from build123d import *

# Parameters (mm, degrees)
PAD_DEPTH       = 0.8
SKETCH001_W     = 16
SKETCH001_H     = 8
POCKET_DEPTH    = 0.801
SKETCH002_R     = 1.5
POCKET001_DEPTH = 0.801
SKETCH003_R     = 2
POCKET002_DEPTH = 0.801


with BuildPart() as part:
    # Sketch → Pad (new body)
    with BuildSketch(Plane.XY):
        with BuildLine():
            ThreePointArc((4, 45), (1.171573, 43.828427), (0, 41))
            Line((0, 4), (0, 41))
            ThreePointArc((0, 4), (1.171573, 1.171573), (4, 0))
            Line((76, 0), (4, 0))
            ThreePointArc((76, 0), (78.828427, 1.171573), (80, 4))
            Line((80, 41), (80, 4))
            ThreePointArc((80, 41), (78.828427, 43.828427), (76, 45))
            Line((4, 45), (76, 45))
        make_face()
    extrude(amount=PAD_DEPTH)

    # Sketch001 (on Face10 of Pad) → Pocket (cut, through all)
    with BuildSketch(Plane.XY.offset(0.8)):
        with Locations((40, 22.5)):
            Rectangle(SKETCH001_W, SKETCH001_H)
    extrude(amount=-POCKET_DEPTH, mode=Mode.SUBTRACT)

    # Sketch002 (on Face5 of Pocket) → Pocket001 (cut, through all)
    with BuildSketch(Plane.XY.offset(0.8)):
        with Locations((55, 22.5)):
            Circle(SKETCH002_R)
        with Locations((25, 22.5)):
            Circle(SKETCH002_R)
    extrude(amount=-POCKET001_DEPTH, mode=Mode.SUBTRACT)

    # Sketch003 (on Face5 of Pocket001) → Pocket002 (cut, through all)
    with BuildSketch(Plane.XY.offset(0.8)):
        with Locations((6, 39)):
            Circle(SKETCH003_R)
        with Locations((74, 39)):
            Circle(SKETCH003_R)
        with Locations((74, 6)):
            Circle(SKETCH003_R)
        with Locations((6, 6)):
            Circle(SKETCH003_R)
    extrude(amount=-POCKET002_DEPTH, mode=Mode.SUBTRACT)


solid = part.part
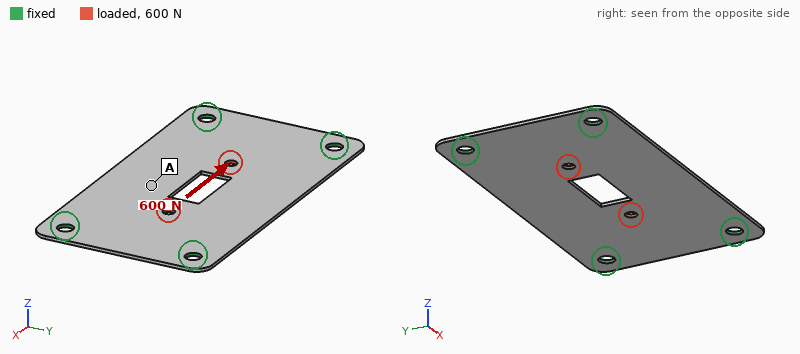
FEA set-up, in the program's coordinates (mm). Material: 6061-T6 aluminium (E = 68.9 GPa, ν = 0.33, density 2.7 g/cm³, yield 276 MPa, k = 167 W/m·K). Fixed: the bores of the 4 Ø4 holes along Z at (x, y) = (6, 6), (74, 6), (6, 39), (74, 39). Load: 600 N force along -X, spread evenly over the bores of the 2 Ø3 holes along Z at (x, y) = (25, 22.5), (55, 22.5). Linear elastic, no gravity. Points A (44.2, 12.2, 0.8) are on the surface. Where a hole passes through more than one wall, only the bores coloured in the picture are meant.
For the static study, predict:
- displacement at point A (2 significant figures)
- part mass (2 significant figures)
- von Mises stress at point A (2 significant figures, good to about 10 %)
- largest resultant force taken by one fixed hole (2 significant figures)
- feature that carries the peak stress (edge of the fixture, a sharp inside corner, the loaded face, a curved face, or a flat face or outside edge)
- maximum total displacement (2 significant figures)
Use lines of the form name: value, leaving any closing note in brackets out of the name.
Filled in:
displacement at point A: 3.6 µm
part mass: 7.3 g
von Mises stress at point A: 7.7 MPa
largest resultant force taken by one fixed hole: 160 N
feature that carries the peak stress: the loaded face
maximum total displacement: 7.7 µm
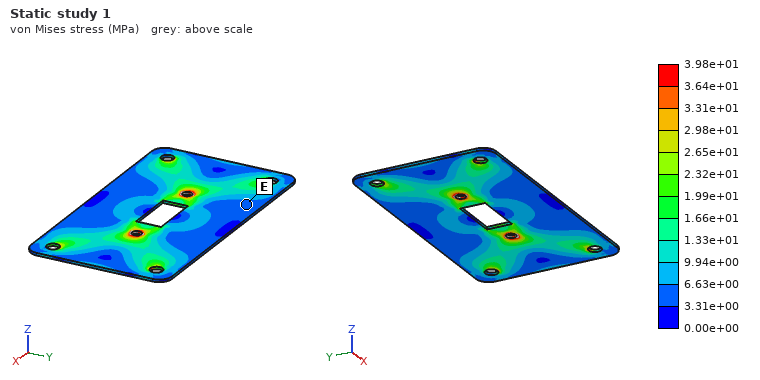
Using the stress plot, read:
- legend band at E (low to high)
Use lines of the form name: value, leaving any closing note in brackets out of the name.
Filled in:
legend band at E: 3.31e+00 to 6.63e+00 MPa
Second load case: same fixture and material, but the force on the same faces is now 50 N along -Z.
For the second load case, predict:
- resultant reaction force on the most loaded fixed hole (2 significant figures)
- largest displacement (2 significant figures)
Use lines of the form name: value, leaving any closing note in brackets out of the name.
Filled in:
resultant reaction force on the most loaded fixed hole: 13 N
largest displacement: 0.52 mm
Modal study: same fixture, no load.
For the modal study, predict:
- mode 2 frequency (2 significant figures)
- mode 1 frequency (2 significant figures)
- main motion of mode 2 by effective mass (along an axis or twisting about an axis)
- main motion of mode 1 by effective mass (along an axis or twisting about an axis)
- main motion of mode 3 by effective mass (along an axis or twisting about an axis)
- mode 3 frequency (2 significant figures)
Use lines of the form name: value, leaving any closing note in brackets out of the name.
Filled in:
mode 2 frequency: 1300 Hz
mode 1 frequency: 920 Hz
main motion of mode 2 by effective mass: twisting about X
main motion of mode 1 by effective mass: along Z
main motion of mode 3 by effective mass: twisting about Y
mode 3 frequency: 2400 Hz
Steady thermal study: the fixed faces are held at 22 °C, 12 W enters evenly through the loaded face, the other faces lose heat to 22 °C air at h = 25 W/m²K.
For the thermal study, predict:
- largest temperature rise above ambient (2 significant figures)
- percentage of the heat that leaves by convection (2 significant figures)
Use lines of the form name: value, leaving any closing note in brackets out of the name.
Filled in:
largest temperature rise above ambient: 33 K
percentage of the heat that leaves by convection: 18 %
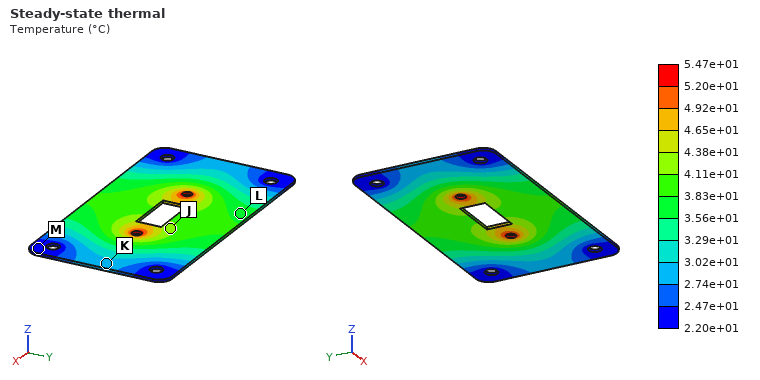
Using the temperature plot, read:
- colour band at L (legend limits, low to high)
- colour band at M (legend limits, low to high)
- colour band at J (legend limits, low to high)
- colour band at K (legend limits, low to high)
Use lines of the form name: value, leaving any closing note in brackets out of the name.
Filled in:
colour band at L: 3.56e+01 to 3.83e+01 °C
colour band at M: 2.20e+01 to 2.47e+01 °C
colour band at J: 4.11e+01 to 4.38e+01 °C
colour band at K: 2.74e+01 to 3.02e+01 °C
